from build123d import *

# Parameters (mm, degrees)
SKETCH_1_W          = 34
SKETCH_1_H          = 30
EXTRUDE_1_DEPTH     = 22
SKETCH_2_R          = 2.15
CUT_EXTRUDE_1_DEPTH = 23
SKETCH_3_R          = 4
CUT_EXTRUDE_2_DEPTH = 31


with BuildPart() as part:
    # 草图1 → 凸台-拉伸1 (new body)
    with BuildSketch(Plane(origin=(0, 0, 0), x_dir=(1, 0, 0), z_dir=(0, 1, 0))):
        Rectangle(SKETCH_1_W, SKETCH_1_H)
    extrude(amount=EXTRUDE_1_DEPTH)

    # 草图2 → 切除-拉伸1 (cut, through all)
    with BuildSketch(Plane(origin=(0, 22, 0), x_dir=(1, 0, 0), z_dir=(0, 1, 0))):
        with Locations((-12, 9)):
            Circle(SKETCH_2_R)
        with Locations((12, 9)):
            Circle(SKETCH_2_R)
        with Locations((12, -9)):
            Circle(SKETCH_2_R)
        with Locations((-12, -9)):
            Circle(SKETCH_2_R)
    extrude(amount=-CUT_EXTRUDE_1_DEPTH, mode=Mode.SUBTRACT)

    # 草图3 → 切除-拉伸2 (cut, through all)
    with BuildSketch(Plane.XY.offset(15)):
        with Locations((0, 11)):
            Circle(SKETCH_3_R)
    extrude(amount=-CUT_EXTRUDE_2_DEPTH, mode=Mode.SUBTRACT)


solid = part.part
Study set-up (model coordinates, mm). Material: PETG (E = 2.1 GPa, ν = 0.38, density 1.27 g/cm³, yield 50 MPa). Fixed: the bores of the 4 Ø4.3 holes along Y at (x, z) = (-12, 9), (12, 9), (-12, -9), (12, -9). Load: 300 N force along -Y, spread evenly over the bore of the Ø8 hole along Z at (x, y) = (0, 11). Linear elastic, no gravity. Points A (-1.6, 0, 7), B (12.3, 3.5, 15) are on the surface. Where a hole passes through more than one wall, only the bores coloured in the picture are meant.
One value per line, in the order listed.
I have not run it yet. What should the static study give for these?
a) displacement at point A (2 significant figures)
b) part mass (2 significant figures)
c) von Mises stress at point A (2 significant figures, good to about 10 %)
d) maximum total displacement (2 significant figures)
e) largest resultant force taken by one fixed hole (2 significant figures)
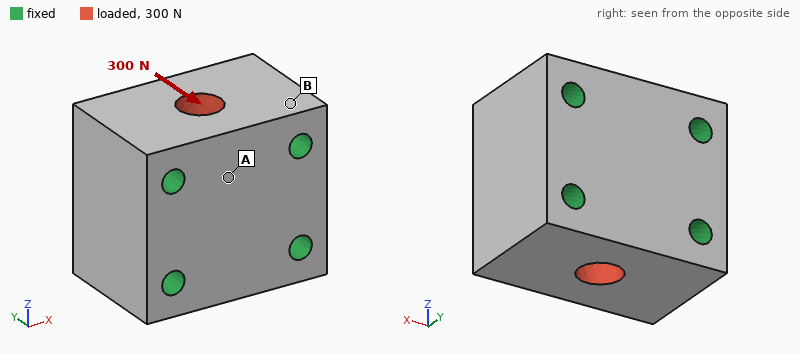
3.1 µm
25 g
0.39 MPa
4.2 µm
75 N
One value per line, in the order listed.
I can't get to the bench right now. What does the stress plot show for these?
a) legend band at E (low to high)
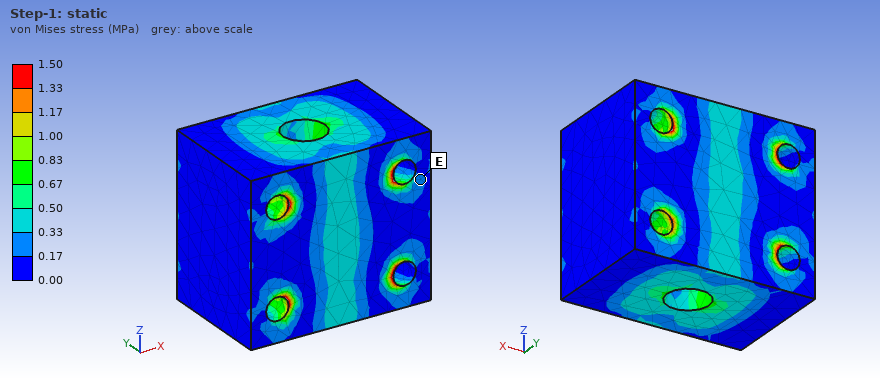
0.17 to 0.33 MPa
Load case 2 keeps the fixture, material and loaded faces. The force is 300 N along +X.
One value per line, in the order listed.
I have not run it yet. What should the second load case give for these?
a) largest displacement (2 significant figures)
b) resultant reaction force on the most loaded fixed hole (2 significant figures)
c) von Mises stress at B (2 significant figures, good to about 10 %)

1.9 µm
76 N
0.11 MPa
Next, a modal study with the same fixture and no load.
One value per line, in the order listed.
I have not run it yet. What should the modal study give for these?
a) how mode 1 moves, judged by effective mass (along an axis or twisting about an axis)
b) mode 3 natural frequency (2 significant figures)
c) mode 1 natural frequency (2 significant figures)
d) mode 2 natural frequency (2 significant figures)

along Y
17 kHz
15 kHz
16 kHz
